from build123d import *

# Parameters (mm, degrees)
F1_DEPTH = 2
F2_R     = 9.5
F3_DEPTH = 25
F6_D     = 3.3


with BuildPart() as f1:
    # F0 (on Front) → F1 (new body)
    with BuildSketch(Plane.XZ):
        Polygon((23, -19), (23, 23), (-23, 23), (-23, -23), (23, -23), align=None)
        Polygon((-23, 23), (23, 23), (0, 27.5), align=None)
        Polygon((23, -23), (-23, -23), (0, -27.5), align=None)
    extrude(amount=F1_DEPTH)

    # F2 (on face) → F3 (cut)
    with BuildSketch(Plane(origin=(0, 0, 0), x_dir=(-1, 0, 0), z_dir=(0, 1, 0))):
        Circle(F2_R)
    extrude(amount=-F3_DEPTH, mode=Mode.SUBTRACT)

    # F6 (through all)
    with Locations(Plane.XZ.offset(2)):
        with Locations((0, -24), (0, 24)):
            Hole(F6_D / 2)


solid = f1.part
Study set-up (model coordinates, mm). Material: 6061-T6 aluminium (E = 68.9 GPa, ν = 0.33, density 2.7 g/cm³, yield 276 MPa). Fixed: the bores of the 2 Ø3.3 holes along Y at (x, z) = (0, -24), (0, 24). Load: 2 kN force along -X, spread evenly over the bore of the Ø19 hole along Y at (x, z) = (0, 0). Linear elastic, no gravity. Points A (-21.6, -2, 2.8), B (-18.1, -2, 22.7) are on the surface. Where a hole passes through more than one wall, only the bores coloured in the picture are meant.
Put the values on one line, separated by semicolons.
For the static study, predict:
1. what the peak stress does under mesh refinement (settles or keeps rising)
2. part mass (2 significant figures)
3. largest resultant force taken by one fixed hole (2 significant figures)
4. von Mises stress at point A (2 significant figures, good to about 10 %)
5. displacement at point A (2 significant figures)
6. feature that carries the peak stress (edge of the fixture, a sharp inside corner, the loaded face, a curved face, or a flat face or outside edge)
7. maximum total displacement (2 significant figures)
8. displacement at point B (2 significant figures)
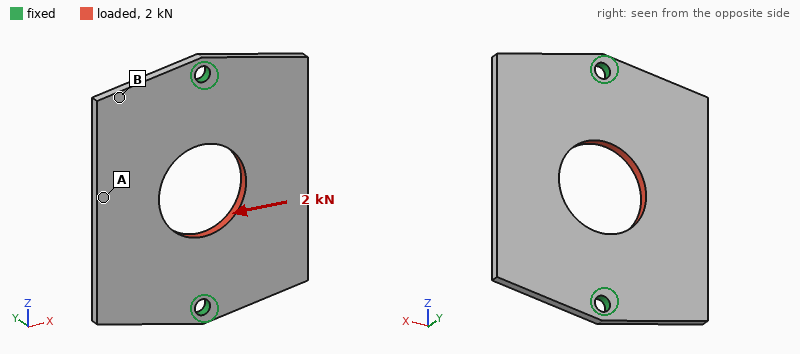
keeps rising; 11 g; 1.0 kN; 29 MPa; 14 µm; edge of the fixture; 16 µm; 6.4 µm
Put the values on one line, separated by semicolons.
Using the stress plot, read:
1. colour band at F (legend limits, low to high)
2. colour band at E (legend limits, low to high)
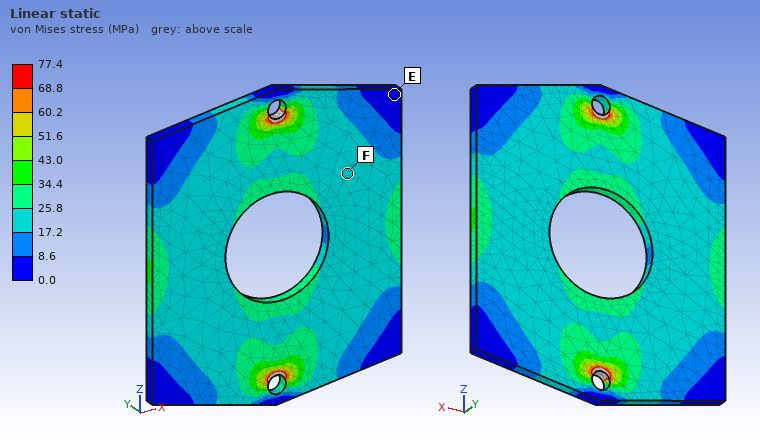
17.2 to 25.8 MPa; 0.0 to 8.6 MPa
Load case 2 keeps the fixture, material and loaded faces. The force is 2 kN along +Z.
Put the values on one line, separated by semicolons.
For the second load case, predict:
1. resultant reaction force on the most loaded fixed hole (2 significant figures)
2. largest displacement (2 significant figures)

1.0 kN; 12 µm
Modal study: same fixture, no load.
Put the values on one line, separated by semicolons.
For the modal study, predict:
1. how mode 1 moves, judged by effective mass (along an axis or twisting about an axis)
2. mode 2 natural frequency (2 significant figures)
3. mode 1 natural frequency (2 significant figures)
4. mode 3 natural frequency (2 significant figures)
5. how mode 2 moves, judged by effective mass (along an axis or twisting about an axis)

twisting about Z; 2500 Hz; 1900 Hz; 4500 Hz; along Y
